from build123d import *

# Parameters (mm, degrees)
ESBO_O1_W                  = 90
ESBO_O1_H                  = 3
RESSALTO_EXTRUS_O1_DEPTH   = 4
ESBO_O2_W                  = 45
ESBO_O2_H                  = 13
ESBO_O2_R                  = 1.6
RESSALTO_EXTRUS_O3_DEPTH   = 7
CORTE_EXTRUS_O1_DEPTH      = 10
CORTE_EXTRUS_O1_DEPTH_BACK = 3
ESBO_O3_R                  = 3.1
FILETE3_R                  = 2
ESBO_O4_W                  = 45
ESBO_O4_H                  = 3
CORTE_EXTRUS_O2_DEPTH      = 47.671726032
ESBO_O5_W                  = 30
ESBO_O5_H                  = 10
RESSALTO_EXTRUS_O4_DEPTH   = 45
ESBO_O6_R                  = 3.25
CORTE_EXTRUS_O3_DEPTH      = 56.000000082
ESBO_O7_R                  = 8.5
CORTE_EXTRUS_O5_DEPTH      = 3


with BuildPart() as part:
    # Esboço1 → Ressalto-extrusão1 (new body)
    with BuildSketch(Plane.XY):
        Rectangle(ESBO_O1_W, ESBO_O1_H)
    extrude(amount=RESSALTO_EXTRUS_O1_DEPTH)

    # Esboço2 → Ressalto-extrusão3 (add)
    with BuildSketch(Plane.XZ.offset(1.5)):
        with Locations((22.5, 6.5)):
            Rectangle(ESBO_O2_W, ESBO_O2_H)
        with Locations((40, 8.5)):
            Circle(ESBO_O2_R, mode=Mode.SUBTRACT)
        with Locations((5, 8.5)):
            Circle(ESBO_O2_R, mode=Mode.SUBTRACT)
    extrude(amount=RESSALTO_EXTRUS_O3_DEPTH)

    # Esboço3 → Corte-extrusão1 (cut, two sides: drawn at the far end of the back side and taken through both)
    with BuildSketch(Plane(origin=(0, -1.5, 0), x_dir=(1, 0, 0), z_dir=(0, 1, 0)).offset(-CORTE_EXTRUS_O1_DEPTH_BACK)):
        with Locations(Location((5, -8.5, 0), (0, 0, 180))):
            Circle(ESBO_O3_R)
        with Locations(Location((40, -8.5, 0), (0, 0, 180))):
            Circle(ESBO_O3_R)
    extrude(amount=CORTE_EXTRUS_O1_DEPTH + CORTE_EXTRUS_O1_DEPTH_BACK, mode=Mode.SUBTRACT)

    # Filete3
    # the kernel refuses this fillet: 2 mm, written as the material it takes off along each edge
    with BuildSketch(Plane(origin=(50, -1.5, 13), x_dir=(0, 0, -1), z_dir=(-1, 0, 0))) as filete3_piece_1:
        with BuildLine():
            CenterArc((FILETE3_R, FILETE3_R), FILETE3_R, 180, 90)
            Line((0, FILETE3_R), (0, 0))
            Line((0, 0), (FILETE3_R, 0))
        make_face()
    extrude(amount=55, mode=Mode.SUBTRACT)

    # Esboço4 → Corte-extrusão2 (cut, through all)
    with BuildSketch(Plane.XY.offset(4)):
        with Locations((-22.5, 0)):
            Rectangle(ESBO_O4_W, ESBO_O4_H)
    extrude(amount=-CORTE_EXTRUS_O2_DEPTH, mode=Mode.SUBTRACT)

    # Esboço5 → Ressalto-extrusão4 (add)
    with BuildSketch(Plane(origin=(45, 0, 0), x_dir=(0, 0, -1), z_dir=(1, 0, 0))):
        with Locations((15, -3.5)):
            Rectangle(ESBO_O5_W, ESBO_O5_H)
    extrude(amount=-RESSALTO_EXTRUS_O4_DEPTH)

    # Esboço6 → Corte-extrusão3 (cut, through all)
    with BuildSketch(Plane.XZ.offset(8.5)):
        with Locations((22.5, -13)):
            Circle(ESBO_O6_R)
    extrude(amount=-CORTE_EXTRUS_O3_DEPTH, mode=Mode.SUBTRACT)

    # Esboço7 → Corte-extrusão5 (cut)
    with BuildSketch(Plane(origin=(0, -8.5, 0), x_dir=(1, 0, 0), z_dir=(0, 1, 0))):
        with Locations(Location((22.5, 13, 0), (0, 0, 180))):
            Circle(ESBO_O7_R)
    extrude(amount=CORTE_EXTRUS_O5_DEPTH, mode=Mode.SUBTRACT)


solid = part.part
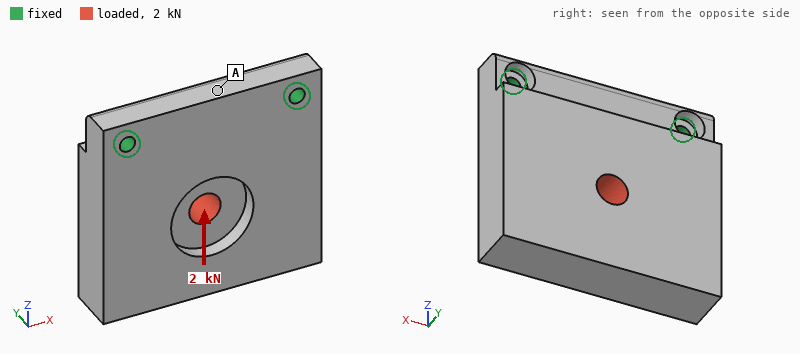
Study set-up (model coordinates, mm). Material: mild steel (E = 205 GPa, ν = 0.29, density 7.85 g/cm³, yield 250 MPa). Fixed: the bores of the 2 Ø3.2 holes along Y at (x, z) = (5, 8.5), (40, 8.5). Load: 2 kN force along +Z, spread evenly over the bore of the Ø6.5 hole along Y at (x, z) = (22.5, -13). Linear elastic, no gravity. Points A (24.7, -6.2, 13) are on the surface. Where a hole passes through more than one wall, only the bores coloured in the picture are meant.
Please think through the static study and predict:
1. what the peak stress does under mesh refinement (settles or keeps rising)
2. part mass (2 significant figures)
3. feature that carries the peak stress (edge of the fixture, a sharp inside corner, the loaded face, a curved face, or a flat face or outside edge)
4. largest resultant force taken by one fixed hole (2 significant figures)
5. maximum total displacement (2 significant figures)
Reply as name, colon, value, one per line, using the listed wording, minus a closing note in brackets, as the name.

what the peak stress does under mesh refinement: keeps rising
part mass: 130 g
feature that carries the peak stress: edge of the fixture
largest resultant force taken by one fixed hole: 1.0 kN
maximum total displacement: 32 µm
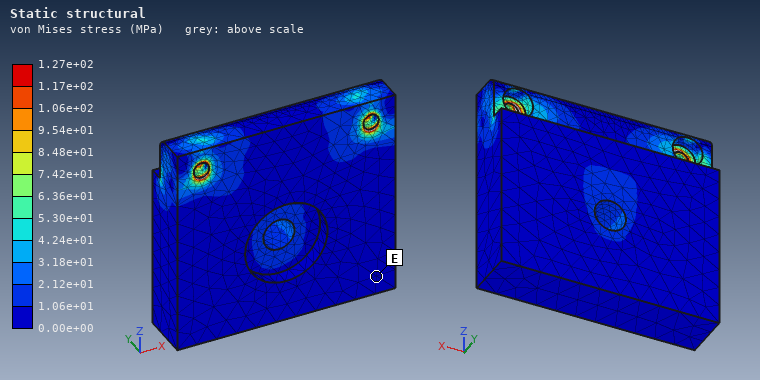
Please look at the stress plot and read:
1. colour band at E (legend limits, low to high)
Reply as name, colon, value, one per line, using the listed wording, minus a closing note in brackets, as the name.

colour band at E: 0.00e+00 to 1.06e+01 MPa
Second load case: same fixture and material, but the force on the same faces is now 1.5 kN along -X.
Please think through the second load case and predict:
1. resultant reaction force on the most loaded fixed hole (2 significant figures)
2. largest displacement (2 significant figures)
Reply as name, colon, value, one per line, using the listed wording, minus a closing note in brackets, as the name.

resultant reaction force on the most loaded fixed hole: 1.2 kN
largest displacement: 3.8 µm
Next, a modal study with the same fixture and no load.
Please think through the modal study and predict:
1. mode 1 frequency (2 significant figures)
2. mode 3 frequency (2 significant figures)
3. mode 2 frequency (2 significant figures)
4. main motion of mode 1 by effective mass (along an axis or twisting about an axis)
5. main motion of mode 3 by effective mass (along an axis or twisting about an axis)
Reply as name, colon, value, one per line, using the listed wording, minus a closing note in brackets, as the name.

mode 1 frequency: 2100 Hz
mode 3 frequency: 11 kHz
mode 2 frequency: 7400 Hz
main motion of mode 1 by effective mass: along Y
main motion of mode 3 by effective mass: along X
